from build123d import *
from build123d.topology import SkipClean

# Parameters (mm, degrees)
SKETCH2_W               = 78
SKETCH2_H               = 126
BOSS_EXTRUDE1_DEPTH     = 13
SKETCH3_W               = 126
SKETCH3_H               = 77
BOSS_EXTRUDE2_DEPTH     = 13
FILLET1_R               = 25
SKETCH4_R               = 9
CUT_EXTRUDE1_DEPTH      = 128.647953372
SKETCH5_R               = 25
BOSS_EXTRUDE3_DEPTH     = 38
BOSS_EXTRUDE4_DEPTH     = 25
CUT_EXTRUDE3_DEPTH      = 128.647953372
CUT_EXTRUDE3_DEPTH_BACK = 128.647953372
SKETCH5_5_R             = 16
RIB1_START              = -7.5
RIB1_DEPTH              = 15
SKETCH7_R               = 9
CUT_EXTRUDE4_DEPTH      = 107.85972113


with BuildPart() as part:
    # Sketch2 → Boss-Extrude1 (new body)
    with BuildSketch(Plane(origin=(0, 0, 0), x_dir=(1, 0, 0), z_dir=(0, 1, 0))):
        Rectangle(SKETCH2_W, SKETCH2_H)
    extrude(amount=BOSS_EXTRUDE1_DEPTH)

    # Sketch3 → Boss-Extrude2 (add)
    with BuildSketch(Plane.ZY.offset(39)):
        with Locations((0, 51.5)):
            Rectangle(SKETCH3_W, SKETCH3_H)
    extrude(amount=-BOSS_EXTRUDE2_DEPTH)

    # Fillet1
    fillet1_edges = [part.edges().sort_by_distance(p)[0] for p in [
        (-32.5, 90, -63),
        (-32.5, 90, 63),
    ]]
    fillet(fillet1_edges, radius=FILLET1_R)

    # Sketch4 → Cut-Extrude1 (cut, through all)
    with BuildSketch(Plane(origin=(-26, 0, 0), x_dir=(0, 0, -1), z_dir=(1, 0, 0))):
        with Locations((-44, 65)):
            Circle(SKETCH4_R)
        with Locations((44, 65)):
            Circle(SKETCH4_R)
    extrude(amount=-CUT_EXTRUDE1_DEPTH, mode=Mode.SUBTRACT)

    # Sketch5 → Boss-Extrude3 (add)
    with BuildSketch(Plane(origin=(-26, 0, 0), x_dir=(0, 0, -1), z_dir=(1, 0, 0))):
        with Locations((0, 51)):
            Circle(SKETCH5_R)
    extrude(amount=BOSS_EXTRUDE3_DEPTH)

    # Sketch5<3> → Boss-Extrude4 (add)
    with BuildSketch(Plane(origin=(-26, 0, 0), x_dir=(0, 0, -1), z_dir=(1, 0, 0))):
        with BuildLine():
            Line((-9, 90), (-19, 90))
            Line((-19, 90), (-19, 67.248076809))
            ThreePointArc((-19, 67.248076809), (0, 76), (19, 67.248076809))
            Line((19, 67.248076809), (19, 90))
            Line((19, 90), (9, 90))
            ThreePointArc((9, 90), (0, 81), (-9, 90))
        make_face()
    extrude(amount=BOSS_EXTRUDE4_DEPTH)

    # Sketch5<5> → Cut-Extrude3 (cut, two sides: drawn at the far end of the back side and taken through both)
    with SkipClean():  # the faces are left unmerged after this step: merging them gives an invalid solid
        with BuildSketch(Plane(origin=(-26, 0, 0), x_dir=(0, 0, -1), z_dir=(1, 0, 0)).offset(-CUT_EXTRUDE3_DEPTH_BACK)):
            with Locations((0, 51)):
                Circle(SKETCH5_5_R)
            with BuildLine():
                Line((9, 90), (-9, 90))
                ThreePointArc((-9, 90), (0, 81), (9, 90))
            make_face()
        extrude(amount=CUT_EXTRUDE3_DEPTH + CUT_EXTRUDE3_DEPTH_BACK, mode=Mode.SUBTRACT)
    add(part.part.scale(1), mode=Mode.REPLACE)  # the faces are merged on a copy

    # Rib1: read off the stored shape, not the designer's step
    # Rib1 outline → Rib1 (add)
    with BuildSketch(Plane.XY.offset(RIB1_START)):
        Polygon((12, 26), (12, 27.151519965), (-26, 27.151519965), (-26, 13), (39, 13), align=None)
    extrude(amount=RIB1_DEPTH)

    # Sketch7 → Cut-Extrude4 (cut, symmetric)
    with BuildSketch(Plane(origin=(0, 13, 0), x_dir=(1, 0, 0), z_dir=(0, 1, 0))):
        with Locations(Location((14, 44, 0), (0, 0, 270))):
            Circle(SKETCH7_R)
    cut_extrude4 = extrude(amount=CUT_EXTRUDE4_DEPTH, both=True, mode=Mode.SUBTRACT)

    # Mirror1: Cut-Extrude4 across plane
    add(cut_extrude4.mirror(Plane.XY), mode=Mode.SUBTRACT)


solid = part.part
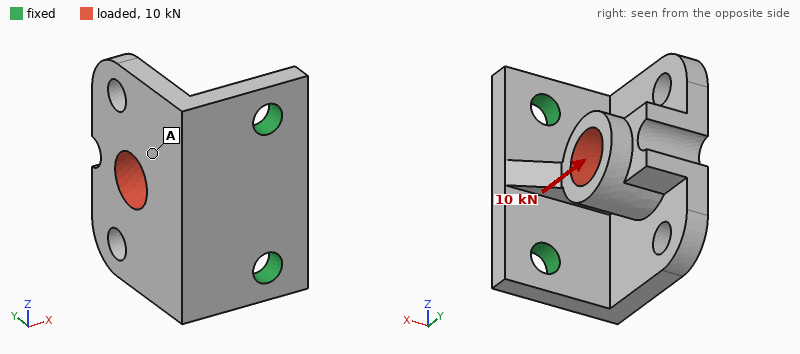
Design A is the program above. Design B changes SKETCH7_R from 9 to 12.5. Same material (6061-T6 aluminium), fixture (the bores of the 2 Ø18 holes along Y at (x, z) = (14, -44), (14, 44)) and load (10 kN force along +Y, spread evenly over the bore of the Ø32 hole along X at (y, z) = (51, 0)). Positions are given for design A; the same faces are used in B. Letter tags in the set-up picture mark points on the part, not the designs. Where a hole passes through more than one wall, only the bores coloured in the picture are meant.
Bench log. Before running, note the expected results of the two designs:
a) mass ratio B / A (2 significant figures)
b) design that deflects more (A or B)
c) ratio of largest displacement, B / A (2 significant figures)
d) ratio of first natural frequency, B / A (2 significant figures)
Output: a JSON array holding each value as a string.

["0.98", "A", "0.67", "1.1"]
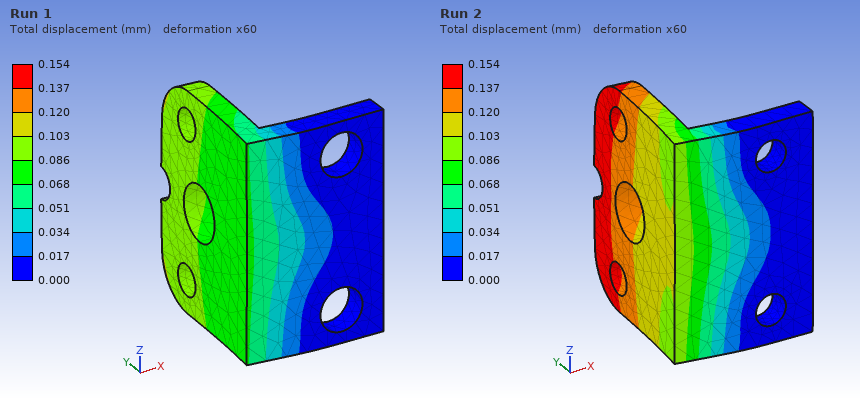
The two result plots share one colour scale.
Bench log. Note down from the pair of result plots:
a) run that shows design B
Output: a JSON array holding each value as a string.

["Run 1"]
